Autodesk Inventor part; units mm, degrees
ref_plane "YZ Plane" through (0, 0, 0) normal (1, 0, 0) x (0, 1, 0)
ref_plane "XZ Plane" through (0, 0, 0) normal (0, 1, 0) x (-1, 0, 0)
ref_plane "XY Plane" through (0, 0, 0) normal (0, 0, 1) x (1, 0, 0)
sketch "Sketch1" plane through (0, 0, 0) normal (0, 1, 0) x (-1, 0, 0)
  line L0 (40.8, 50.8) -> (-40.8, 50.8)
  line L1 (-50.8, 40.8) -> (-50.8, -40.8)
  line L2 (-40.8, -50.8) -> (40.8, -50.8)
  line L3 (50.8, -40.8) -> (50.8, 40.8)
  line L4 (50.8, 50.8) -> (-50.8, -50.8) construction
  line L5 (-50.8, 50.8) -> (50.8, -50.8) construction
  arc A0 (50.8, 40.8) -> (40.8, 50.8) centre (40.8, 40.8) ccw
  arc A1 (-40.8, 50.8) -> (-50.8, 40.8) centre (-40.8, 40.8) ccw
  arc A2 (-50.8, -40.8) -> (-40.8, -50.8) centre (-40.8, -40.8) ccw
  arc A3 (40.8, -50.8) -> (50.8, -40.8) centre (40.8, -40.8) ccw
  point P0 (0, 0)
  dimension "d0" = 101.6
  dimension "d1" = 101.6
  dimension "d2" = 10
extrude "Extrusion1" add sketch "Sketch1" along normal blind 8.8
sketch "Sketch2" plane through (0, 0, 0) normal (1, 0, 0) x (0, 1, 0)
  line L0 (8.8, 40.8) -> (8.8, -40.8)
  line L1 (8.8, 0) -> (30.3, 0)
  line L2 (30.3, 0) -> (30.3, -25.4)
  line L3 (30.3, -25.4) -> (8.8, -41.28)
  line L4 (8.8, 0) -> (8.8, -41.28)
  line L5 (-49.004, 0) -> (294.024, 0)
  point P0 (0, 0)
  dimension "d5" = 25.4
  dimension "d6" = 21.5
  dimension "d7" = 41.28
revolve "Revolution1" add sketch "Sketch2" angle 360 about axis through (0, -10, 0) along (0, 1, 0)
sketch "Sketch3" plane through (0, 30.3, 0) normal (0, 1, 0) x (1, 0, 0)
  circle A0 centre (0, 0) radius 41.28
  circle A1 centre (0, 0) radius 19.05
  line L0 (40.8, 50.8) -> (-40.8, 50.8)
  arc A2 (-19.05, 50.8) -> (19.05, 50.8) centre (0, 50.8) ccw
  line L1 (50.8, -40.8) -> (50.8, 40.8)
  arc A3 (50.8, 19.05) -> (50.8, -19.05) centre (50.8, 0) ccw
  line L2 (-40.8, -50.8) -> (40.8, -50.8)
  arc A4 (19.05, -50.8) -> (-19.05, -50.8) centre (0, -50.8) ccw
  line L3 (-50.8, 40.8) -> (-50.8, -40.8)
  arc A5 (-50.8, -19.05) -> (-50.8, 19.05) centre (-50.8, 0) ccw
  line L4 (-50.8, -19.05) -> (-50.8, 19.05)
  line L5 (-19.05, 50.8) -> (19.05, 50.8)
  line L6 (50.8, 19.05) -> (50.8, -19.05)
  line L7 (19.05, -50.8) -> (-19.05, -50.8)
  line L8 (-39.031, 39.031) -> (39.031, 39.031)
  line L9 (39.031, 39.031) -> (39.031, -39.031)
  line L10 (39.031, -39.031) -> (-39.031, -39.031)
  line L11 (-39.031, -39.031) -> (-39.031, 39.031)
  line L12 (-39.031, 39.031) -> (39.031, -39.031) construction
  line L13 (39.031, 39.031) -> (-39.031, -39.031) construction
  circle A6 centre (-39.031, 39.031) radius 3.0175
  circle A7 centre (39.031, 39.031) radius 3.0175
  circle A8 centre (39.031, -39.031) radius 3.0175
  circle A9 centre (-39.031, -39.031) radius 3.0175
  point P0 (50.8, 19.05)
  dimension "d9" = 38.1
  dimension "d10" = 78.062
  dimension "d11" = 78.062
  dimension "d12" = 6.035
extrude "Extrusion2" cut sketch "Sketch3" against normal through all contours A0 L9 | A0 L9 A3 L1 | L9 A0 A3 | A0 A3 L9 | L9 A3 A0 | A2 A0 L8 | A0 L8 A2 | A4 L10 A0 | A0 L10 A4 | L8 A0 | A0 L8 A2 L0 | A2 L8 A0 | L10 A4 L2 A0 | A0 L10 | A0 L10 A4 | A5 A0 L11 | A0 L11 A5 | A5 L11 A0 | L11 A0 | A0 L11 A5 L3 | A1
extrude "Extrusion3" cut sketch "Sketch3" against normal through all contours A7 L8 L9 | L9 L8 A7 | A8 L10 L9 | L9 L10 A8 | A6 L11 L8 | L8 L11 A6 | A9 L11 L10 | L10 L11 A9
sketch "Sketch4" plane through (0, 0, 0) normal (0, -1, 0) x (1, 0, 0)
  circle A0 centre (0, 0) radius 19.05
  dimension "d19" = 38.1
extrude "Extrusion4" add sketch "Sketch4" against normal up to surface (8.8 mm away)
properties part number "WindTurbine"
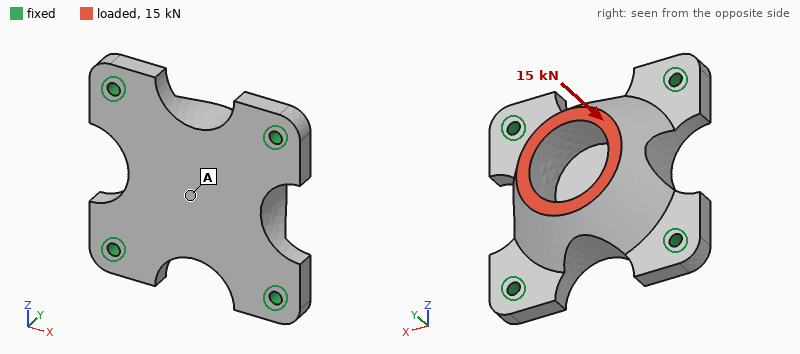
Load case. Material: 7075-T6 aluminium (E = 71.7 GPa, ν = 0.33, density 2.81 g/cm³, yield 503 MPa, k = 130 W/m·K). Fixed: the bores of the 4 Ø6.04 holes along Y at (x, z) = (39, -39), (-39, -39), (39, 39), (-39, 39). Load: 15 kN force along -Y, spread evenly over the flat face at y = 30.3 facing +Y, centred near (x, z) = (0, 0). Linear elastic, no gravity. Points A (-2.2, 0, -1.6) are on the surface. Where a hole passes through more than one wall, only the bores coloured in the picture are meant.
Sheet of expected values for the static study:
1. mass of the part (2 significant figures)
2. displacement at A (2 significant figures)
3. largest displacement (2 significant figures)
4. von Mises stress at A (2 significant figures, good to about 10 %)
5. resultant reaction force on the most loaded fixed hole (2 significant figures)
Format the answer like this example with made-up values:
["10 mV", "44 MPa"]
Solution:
["330 g", "49 µm", "49 µm", "13 MPa", "4.5 kN"]
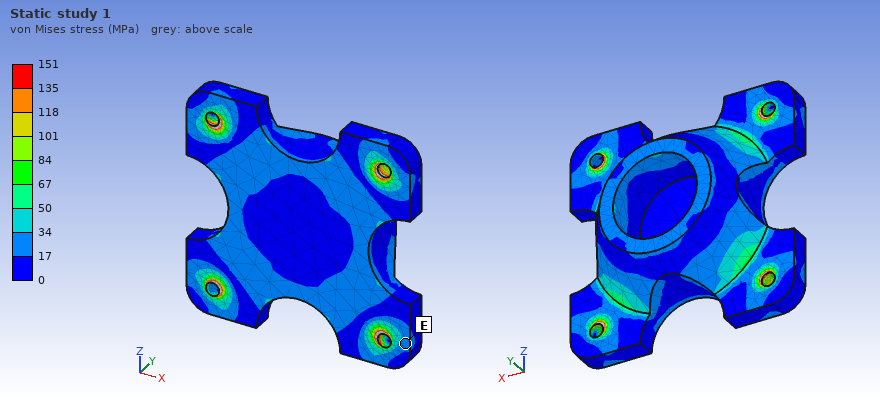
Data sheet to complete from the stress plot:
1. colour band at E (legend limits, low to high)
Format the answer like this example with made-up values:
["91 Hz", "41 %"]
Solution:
["17 to 34 MPa"]
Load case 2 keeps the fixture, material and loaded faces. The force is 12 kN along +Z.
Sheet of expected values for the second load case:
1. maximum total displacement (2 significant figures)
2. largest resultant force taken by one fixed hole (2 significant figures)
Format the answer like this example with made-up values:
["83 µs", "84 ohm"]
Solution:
["39 µm", "4.2 kN"]
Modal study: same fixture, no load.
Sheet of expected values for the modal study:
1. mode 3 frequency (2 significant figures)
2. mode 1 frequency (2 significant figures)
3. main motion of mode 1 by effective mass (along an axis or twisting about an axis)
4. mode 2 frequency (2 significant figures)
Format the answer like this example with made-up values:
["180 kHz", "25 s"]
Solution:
["8900 Hz", "5800 Hz", "along Y", "8900 Hz"]
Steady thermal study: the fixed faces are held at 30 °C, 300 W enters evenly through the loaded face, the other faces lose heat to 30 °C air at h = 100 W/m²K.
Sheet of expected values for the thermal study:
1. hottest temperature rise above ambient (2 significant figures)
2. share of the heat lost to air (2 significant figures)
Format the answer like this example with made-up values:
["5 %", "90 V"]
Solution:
["69 K", "25 %"]
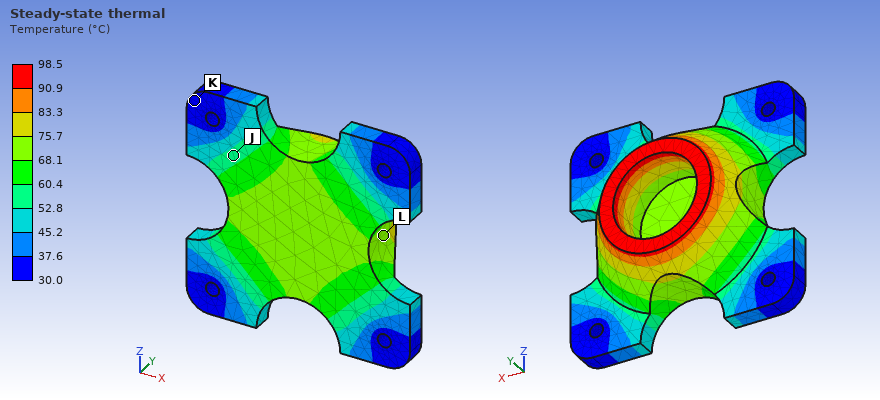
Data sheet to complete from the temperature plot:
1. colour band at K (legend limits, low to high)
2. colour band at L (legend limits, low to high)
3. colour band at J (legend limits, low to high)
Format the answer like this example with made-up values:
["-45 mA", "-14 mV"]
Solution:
["30.0 to 37.6 °C", "68.1 to 75.7 °C", "52.8 to 60.4 °C"]
